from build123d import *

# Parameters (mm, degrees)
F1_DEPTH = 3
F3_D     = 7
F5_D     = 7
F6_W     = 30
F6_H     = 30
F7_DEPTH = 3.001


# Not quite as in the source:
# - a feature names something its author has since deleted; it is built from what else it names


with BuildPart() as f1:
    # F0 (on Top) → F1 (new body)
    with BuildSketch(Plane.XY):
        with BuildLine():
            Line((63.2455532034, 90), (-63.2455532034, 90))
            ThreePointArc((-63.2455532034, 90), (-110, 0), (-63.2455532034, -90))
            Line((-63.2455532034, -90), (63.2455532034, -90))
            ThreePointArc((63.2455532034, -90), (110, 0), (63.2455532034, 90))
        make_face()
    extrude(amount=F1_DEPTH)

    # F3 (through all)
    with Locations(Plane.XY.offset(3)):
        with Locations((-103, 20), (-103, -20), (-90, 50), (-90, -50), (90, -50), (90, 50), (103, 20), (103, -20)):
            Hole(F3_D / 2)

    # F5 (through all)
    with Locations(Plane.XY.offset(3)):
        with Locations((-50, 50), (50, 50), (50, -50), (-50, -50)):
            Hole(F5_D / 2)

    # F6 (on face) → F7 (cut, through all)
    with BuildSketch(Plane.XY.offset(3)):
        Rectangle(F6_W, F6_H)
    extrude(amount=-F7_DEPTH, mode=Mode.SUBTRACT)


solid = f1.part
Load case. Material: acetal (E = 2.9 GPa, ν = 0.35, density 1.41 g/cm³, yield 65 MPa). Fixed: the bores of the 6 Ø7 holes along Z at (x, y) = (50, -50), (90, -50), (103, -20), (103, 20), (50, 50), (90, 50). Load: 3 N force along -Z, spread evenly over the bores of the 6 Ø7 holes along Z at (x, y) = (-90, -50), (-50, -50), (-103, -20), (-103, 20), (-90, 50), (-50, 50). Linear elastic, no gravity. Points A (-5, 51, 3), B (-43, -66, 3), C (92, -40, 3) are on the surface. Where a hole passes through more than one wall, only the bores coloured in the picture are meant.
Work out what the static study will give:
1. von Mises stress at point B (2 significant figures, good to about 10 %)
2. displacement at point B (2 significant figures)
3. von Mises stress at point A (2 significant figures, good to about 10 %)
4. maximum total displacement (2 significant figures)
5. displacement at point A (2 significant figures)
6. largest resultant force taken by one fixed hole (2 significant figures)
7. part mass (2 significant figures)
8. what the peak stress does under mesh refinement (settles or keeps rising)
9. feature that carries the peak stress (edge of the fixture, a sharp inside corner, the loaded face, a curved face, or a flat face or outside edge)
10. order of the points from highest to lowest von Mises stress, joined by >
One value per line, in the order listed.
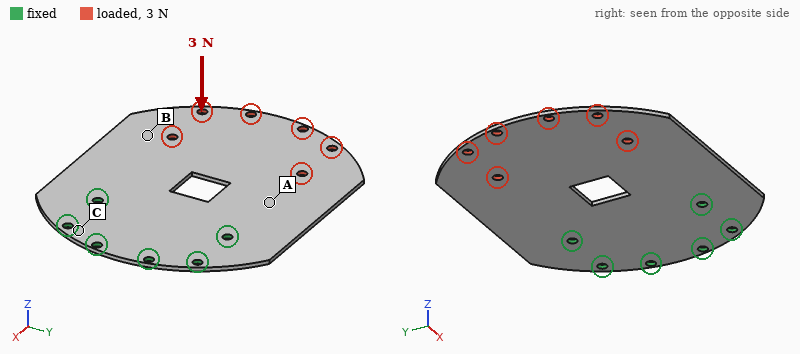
0.47 MPa
1.2 mm
0.92 MPa
2.9 mm
0.50 mm
3.6 N
140 g
keeps rising
edge of the fixture
A > B > C
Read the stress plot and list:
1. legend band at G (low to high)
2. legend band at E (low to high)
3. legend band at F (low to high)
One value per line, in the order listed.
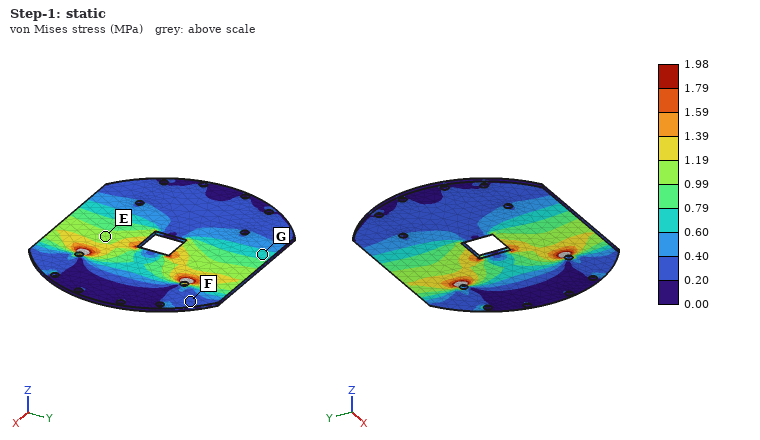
0.60 to 0.79 MPa
0.99 to 1.19 MPa
0.20 to 0.40 MPa
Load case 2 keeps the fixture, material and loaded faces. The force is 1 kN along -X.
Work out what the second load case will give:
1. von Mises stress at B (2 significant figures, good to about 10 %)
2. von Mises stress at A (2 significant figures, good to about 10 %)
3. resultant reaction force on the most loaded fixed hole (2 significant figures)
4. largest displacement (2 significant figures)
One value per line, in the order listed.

1.9 MPa
2.3 MPa
340 N
0.16 mm
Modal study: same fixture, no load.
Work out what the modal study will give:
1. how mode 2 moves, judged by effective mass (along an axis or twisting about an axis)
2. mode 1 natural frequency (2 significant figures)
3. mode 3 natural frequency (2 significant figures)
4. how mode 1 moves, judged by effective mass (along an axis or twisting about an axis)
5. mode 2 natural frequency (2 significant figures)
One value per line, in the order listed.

twisting about X
30 Hz
160 Hz
along Z
73 Hz
